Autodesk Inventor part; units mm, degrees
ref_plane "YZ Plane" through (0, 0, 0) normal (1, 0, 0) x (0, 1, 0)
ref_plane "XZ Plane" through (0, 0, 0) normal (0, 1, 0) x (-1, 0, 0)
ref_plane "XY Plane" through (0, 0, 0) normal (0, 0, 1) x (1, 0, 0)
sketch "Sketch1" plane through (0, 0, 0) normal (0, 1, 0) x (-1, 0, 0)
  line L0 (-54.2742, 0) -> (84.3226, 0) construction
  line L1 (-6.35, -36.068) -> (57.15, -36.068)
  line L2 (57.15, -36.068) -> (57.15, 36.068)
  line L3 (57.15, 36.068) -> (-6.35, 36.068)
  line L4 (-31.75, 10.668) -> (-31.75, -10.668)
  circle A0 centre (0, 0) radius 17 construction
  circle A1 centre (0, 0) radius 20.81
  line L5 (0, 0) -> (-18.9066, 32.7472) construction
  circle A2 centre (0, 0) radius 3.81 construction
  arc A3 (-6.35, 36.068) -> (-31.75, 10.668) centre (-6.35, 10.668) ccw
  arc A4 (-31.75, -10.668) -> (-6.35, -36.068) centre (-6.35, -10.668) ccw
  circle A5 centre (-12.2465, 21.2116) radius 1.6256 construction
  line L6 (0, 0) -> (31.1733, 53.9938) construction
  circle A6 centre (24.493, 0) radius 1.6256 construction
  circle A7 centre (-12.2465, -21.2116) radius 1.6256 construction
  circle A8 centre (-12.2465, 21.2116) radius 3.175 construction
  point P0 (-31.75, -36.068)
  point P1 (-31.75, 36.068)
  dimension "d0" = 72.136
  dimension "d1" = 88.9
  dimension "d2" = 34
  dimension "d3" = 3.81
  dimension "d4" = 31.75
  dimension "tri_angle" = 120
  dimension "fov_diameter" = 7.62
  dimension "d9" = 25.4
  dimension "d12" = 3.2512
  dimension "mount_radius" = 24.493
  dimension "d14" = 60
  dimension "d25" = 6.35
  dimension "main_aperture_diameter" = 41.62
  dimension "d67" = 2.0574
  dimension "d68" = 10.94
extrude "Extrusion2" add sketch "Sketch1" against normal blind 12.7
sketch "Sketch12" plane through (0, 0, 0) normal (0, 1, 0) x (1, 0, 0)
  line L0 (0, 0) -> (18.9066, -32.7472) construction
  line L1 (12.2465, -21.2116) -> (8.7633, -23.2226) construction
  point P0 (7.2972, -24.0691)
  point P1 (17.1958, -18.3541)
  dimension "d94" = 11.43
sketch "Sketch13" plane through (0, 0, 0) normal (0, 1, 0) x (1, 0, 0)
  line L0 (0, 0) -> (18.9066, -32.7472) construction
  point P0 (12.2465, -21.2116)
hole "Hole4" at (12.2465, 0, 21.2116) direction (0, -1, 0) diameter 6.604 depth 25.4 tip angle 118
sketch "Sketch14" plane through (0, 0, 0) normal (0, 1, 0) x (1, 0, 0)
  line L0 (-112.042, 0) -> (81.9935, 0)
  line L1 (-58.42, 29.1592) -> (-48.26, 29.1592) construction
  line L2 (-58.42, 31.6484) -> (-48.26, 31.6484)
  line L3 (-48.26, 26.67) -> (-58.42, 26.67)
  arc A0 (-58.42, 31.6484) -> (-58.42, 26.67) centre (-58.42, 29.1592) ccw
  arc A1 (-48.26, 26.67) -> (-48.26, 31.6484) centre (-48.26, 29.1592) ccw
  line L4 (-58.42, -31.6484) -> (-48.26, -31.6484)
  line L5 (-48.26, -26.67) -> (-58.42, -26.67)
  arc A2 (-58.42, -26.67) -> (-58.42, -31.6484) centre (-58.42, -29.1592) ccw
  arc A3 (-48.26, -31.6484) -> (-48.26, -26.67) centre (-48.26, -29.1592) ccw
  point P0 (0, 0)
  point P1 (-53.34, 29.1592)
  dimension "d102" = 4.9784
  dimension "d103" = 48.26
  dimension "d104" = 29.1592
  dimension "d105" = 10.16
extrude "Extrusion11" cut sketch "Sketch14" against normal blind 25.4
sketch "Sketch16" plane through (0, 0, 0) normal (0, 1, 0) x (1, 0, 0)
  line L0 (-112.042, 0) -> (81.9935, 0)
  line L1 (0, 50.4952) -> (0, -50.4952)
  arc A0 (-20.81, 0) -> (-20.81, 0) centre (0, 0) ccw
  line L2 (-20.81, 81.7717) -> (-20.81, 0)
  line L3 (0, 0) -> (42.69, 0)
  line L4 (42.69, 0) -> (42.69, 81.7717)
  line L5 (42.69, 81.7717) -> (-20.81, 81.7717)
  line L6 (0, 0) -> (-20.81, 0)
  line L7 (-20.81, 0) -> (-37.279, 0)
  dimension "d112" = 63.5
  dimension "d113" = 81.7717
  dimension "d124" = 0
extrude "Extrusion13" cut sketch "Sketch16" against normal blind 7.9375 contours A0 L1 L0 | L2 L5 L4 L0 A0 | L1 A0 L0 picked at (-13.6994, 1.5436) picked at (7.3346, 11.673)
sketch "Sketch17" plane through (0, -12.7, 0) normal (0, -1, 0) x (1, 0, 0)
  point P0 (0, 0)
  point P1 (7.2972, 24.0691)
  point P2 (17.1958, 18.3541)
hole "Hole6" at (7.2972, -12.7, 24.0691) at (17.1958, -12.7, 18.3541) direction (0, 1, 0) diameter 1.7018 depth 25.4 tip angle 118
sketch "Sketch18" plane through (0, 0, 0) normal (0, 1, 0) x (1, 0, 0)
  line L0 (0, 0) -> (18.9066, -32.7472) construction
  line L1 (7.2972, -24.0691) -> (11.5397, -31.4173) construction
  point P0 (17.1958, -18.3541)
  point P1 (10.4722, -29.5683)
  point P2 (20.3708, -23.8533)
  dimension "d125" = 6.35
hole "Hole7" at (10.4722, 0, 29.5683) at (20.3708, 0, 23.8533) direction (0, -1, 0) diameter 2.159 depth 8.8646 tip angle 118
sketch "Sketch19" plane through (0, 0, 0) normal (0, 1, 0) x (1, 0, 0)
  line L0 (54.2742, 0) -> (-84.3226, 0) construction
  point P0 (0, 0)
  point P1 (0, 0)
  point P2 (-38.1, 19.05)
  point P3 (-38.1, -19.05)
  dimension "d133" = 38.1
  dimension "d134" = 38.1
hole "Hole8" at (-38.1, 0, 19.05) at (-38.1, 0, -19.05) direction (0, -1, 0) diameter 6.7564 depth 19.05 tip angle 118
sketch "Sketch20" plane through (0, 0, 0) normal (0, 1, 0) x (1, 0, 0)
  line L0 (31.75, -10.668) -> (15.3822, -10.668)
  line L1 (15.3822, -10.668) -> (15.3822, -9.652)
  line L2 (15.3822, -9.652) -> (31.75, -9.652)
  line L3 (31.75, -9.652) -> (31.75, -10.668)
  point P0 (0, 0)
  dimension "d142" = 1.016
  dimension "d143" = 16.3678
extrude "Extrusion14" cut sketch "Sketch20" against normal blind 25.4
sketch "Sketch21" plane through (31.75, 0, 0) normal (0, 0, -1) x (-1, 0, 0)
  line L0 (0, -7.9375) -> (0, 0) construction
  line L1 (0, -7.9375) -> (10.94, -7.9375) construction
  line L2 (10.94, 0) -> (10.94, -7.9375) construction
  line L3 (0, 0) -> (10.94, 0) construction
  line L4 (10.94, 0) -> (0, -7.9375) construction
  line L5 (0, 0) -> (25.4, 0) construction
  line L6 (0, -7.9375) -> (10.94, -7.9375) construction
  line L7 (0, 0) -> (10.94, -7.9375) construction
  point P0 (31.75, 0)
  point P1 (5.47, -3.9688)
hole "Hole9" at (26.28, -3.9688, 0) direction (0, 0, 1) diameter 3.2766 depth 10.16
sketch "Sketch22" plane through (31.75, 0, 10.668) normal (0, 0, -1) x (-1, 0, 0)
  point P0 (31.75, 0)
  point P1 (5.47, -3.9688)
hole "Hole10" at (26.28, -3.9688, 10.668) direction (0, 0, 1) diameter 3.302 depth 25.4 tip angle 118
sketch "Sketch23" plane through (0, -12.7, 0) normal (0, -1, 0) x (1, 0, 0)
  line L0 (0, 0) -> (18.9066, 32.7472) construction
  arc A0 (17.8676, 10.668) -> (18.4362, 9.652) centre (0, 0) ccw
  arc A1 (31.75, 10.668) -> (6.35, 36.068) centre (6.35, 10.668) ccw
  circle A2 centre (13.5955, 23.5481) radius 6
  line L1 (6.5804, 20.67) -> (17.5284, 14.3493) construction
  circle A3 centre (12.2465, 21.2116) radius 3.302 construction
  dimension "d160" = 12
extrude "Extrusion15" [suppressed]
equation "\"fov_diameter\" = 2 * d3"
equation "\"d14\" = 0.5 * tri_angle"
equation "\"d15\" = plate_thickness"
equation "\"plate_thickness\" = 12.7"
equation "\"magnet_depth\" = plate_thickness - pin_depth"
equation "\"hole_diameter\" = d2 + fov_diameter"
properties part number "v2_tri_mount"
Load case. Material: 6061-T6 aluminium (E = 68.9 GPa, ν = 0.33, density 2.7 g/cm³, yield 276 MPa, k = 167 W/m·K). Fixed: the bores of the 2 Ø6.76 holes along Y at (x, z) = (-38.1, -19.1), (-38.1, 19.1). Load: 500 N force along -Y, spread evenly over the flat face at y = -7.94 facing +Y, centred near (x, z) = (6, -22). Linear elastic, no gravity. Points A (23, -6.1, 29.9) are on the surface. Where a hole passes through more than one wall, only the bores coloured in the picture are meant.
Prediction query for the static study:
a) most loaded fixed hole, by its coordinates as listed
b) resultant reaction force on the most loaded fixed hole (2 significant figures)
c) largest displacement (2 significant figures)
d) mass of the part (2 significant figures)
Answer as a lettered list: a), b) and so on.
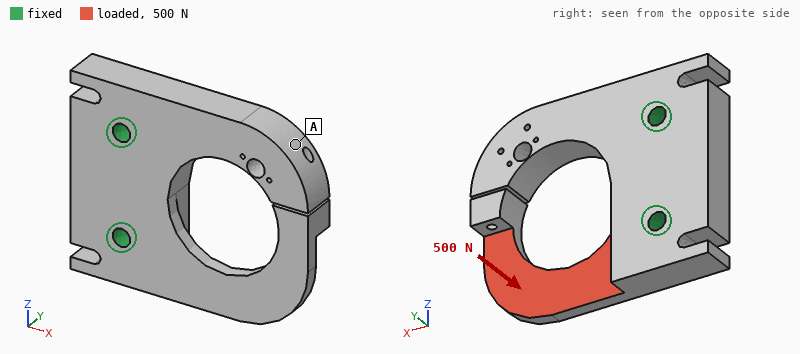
a) (-38.1, -19.1)
b) 540 N
c) 1.2 mm
d) 130 g
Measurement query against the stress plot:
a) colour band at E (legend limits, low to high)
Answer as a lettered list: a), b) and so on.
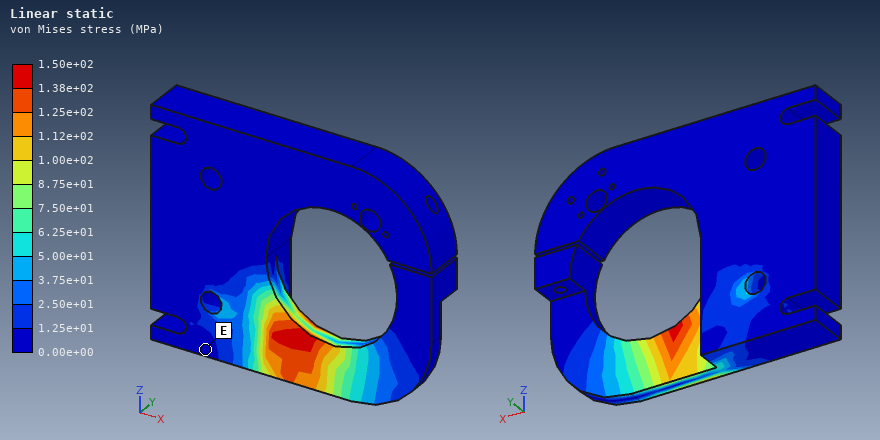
a) 0.00e+00 to 1.25e+01 MPa
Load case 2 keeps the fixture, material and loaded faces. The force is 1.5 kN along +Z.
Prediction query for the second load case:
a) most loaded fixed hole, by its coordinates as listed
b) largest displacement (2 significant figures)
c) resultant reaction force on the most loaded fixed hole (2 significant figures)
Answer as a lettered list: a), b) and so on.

a) (-38.1, 19.1)
b) 0.50 mm
c) 1.7 kN
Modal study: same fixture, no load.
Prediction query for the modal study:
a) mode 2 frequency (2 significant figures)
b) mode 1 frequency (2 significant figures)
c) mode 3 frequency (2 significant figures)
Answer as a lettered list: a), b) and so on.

a) 2100 Hz
b) 760 Hz
c) 2600 Hz
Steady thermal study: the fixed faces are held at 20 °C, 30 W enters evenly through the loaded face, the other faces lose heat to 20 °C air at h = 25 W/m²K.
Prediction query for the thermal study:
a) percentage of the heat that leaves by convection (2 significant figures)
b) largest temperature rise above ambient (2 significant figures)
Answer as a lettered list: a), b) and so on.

a) 12 %
b) 63 K
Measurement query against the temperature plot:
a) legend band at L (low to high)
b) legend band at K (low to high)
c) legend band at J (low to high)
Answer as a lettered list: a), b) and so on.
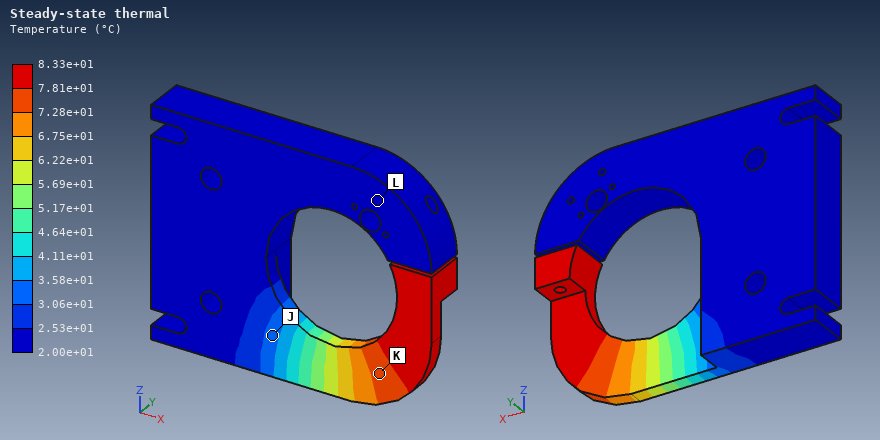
a) 2.00e+01 to 2.53e+01 °C
b) 7.28e+01 to 7.81e+01 °C
c) 3.06e+01 to 3.58e+01 °C
